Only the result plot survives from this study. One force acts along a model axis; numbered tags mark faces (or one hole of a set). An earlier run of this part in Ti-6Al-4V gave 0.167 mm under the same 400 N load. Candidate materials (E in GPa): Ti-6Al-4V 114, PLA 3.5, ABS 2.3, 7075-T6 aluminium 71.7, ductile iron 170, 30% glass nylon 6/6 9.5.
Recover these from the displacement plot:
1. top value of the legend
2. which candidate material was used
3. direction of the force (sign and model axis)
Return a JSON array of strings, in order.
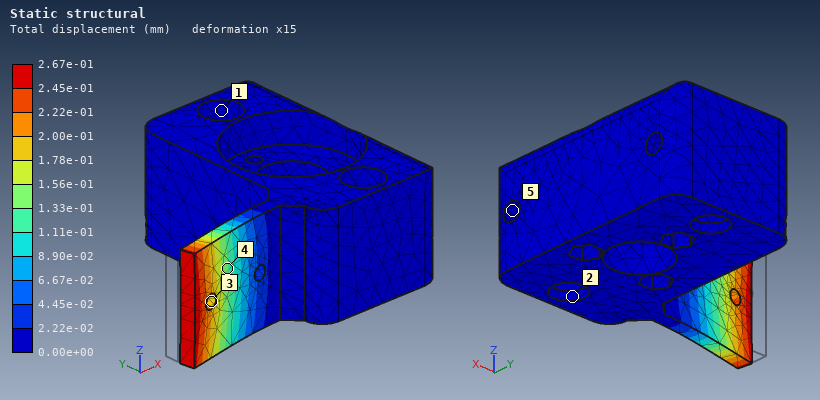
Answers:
["2.67e-01 mm", "7075-T6 aluminium", "-Y"]
